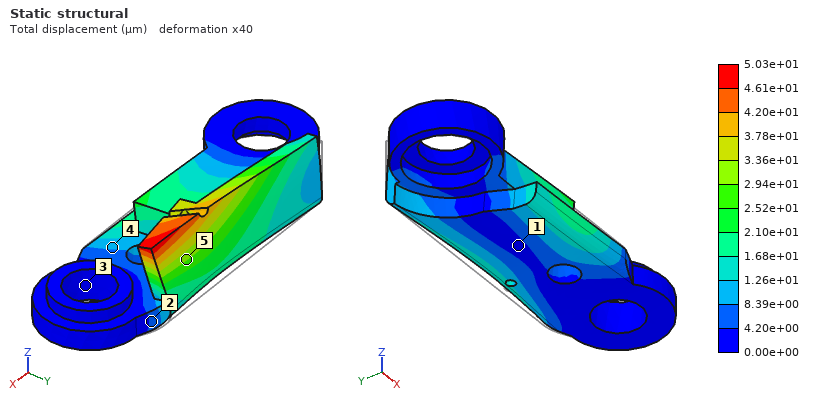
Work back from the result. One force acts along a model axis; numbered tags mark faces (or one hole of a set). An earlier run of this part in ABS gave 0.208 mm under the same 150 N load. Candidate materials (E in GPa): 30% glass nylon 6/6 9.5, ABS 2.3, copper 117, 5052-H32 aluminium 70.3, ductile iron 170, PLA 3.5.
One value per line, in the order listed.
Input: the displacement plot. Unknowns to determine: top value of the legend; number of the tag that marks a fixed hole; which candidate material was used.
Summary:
5.03e+01 µm
3
30% glass nylon 6/6
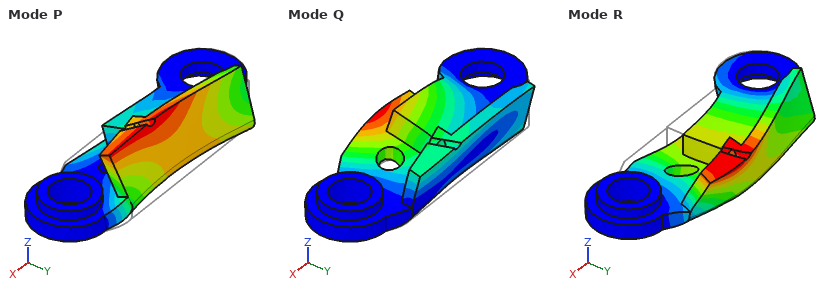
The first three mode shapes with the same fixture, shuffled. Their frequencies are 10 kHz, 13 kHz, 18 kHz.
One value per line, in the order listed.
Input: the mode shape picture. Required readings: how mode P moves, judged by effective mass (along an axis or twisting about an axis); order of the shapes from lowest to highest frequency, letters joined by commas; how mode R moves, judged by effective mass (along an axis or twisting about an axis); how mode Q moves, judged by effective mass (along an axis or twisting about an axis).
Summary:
along Z
P, Q, R
along Y
along Z
